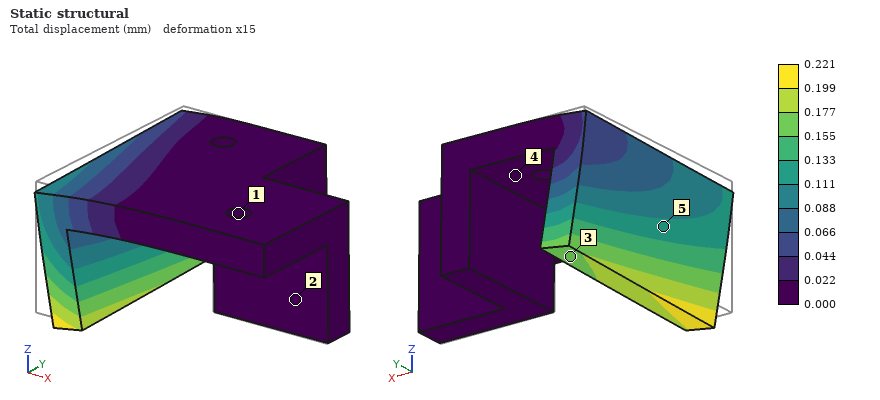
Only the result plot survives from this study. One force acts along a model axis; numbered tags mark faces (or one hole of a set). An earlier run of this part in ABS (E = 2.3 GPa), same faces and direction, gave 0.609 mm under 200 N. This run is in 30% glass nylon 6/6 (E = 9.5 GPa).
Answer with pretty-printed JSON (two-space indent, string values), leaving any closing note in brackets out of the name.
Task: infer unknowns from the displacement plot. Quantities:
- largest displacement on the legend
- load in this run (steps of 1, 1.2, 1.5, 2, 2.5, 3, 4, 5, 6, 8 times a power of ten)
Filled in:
{
  "largest displacement on the legend": "0.221 mm",
  "load in this run": "300 N"
}
